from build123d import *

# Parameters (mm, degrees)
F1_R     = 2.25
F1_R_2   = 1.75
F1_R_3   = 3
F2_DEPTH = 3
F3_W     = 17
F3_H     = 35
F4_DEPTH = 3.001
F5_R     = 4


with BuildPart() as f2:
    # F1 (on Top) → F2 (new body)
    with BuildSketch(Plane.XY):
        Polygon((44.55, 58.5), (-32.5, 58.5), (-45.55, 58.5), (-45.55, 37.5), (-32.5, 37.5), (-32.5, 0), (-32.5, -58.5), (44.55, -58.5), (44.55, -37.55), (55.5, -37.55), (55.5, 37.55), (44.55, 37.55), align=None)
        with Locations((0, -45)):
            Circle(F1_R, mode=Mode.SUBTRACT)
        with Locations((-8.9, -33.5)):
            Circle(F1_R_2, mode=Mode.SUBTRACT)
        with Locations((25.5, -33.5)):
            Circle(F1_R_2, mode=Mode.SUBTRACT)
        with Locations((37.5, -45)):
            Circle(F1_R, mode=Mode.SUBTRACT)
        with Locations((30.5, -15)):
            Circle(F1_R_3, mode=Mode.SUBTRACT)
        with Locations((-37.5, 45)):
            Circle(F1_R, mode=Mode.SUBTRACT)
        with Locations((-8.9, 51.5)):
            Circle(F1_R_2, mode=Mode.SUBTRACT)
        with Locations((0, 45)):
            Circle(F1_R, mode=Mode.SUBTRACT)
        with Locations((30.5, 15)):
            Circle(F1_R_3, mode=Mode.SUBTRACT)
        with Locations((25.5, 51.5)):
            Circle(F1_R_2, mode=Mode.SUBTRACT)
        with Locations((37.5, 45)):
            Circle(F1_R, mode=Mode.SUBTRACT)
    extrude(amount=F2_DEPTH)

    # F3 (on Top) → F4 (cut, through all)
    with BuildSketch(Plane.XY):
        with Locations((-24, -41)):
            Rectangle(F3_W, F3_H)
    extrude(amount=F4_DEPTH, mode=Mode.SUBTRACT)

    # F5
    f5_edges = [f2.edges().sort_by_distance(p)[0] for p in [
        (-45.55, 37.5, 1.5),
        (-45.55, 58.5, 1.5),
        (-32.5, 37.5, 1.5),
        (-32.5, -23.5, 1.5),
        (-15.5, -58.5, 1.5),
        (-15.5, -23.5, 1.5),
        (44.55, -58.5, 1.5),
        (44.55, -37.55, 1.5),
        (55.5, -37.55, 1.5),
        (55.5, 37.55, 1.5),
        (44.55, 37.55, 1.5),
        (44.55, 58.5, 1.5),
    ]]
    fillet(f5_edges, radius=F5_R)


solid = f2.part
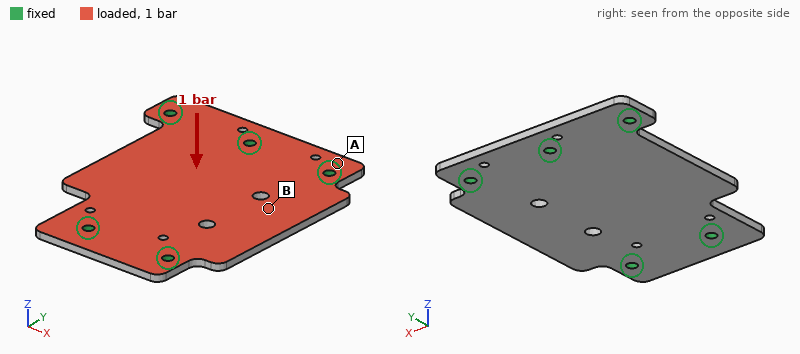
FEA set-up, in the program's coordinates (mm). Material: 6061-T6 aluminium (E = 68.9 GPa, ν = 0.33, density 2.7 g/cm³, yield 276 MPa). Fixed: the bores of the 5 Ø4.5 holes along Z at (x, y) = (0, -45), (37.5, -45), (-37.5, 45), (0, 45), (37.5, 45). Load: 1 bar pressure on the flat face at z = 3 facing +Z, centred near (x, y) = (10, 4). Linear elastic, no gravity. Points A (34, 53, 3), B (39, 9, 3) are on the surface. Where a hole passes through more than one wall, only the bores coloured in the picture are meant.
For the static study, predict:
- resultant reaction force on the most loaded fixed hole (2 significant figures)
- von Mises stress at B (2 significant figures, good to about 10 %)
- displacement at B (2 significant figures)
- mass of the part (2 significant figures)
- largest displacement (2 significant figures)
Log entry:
230 N
22 MPa
0.12 mm
76 g
0.18 mm
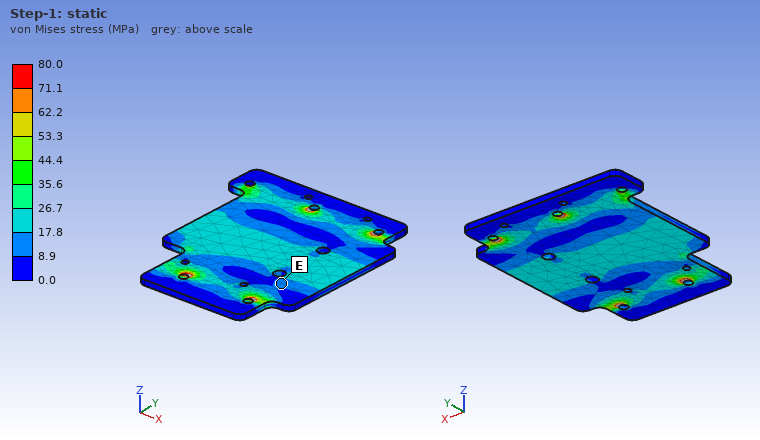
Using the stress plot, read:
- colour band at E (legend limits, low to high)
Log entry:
8.9 to 17.8 MPa
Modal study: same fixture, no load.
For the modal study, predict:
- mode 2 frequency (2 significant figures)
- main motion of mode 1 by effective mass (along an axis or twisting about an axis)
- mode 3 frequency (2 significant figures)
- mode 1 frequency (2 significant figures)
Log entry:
1900 Hz
along Z
3300 Hz
1700 Hz
